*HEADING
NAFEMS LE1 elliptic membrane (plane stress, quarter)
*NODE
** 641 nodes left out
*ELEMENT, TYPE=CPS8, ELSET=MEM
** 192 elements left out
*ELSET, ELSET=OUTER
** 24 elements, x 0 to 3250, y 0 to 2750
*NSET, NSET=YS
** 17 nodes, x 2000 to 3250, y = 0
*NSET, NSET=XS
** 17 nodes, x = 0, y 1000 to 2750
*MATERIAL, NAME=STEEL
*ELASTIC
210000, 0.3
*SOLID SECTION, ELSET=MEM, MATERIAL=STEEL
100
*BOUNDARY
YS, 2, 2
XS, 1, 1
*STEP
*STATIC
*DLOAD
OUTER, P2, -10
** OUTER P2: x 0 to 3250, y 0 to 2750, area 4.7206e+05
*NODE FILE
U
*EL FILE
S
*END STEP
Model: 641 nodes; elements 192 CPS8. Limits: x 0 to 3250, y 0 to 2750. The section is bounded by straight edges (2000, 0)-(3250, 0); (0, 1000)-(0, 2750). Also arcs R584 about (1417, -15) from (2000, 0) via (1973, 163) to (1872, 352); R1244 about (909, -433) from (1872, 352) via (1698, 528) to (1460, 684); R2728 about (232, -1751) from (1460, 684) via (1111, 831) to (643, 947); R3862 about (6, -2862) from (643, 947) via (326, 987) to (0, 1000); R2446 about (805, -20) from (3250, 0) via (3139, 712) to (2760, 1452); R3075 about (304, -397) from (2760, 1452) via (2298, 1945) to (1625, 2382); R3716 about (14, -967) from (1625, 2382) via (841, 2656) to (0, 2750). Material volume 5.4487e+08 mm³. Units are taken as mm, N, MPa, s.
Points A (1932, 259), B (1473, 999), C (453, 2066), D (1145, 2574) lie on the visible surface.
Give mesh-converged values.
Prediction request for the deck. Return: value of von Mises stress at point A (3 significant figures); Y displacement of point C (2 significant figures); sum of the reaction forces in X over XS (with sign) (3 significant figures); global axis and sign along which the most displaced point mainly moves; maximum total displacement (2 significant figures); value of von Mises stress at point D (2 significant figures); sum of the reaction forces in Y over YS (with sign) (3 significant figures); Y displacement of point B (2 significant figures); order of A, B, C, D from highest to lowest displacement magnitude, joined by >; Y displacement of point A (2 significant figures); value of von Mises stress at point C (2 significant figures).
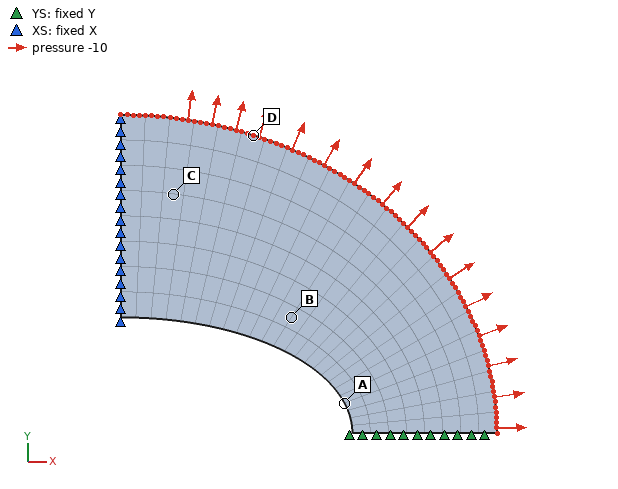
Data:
71.5 MPa
0.53 mm
-2.75e+06 N
+Y
0.55 mm
26 MPa
-3.25e+06 N
0.34 mm
C > D > B > A
0.12 mm
19 MPa
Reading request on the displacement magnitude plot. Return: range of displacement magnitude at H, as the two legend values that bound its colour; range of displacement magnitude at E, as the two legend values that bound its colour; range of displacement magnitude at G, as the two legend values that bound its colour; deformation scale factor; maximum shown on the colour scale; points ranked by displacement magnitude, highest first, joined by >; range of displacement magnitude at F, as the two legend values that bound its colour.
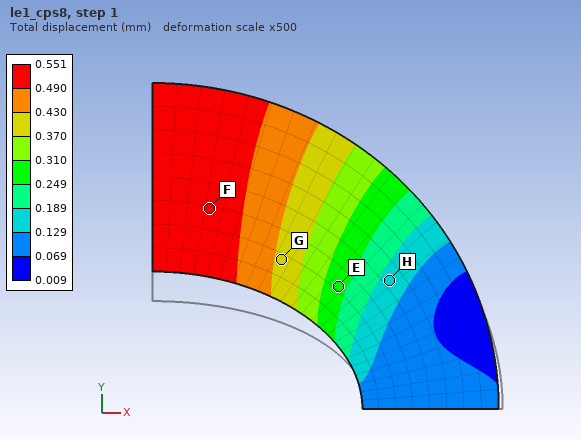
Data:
0.129 to 0.189 mm
0.249 to 0.310 mm
0.370 to 0.430 mm
500
0.551 mm
F > G > E > H
0.490 to 0.551 mm
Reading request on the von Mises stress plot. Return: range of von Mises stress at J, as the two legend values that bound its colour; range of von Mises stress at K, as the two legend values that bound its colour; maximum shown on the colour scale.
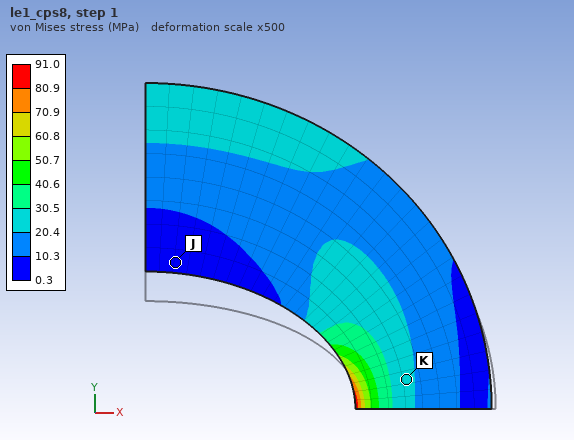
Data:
0.3 to 10.3 MPa
20.4 to 30.5 MPa
91.0 MPa
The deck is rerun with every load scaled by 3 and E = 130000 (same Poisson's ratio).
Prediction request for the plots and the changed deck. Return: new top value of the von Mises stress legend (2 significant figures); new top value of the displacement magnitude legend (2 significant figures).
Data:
270 MPa
2.7 mm
